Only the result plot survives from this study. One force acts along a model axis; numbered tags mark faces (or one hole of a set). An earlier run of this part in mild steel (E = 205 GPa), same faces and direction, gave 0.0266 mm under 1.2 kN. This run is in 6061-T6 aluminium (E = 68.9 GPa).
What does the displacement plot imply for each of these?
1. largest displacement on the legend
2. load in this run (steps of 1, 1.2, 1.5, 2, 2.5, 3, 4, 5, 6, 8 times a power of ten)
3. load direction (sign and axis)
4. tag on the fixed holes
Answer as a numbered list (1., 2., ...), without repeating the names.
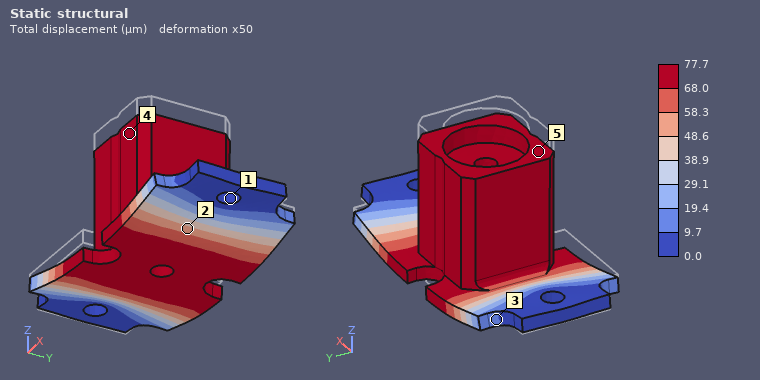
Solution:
1. 77.7 µm
2. 1.2 kN
3. -Z
4. 1
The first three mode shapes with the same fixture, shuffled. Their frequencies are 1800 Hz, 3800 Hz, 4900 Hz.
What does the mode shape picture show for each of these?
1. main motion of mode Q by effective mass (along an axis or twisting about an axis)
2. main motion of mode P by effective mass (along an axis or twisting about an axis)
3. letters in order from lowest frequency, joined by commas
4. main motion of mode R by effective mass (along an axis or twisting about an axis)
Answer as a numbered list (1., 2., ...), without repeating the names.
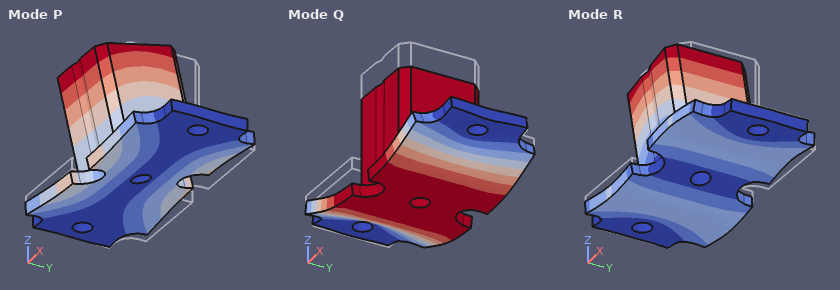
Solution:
1. along Z
2. along Y
3. P, Q, R
4. along X
